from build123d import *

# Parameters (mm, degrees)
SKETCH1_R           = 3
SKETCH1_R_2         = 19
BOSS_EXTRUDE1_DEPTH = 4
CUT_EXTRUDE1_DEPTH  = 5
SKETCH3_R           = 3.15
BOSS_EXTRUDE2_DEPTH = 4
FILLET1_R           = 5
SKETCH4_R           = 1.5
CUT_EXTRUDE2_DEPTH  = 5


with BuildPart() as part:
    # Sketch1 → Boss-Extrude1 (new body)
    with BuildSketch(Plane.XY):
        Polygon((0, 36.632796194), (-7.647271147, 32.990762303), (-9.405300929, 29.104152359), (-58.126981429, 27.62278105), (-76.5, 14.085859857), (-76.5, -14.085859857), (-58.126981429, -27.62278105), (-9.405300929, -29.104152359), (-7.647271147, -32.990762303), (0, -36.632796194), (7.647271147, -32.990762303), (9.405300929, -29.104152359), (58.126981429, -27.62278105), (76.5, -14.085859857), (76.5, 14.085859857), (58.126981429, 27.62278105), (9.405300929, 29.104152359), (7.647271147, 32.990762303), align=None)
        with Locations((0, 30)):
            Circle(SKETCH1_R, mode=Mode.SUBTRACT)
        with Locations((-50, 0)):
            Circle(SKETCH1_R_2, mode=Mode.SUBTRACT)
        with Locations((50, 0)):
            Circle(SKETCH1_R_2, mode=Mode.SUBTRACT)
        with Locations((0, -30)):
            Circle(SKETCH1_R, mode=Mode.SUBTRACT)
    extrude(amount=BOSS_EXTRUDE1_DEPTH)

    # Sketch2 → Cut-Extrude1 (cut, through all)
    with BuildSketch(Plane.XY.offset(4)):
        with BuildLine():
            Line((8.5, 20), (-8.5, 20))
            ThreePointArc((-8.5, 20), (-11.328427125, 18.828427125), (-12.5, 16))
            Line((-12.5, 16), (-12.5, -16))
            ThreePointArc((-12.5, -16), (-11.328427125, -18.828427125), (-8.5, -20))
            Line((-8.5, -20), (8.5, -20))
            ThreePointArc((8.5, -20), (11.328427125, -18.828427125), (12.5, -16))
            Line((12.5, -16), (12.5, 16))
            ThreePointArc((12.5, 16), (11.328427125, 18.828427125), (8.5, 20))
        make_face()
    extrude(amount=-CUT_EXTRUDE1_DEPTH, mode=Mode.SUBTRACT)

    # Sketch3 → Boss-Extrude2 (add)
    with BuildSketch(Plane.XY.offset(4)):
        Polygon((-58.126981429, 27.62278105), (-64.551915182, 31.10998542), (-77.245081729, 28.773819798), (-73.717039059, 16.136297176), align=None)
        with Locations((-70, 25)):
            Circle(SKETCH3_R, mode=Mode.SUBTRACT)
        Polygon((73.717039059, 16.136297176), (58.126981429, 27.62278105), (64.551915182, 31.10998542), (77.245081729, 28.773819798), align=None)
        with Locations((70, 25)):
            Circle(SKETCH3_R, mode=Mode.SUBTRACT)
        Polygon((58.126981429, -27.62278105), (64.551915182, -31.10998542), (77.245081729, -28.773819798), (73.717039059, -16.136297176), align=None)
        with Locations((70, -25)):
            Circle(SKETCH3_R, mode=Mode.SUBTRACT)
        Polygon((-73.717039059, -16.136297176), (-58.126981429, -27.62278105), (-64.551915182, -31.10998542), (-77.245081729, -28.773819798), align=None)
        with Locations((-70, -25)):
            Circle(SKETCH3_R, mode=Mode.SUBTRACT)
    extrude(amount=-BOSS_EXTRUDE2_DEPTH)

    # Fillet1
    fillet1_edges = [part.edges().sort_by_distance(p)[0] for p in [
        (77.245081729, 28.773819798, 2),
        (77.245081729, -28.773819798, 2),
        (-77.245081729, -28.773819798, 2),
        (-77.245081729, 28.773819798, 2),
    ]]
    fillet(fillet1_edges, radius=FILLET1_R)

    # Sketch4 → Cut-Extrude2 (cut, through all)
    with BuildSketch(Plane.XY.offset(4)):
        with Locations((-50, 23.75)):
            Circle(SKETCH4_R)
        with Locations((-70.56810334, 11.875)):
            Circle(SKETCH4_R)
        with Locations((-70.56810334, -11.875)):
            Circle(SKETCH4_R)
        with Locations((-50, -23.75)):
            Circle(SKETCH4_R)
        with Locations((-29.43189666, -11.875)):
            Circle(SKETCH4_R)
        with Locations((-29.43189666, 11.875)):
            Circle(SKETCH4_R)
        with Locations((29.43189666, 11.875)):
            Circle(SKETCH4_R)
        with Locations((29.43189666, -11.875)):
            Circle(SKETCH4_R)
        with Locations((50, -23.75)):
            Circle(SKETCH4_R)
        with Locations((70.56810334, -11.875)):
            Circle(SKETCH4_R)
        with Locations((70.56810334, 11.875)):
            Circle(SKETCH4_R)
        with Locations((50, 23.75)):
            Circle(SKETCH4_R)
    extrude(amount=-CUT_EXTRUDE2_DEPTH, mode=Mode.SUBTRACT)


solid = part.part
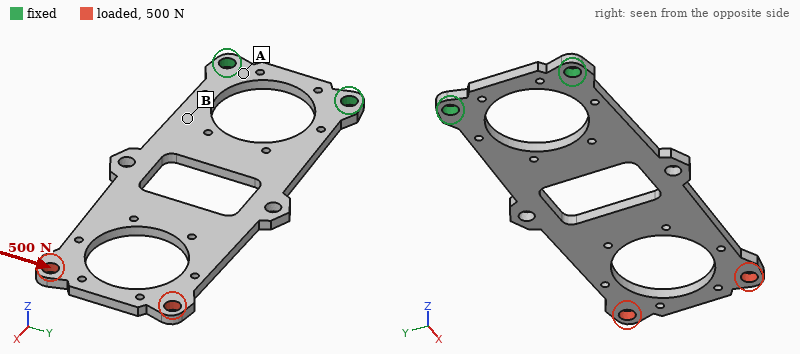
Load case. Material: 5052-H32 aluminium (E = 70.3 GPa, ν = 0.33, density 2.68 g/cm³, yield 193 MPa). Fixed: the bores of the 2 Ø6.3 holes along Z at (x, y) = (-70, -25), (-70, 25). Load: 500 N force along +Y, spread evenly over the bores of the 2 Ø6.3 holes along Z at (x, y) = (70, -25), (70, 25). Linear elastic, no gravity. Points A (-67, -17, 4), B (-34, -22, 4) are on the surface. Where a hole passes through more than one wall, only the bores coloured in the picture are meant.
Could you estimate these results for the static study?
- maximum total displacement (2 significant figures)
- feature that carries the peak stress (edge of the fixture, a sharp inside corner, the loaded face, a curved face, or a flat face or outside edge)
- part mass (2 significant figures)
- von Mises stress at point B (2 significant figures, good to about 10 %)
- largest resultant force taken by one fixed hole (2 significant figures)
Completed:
0.30 mm
a curved face
58 g
21 MPa
1.3 kN
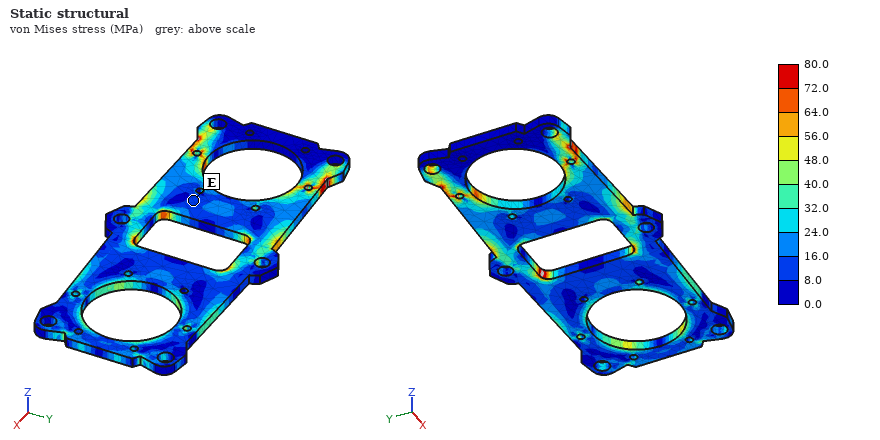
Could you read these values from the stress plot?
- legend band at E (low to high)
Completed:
8.0 to 16.0 MPa
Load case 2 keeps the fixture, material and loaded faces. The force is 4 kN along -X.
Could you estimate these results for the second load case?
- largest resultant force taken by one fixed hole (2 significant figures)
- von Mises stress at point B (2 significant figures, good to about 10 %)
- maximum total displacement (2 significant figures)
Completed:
2.0 kN
39 MPa
0.11 mm
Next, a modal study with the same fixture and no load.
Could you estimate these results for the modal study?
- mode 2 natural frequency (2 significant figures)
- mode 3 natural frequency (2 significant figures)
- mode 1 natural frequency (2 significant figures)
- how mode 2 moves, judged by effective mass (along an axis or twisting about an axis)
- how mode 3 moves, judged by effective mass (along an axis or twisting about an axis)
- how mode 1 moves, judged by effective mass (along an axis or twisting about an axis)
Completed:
650 Hz
770 Hz
130 Hz
twisting about X
along Z
along Z
